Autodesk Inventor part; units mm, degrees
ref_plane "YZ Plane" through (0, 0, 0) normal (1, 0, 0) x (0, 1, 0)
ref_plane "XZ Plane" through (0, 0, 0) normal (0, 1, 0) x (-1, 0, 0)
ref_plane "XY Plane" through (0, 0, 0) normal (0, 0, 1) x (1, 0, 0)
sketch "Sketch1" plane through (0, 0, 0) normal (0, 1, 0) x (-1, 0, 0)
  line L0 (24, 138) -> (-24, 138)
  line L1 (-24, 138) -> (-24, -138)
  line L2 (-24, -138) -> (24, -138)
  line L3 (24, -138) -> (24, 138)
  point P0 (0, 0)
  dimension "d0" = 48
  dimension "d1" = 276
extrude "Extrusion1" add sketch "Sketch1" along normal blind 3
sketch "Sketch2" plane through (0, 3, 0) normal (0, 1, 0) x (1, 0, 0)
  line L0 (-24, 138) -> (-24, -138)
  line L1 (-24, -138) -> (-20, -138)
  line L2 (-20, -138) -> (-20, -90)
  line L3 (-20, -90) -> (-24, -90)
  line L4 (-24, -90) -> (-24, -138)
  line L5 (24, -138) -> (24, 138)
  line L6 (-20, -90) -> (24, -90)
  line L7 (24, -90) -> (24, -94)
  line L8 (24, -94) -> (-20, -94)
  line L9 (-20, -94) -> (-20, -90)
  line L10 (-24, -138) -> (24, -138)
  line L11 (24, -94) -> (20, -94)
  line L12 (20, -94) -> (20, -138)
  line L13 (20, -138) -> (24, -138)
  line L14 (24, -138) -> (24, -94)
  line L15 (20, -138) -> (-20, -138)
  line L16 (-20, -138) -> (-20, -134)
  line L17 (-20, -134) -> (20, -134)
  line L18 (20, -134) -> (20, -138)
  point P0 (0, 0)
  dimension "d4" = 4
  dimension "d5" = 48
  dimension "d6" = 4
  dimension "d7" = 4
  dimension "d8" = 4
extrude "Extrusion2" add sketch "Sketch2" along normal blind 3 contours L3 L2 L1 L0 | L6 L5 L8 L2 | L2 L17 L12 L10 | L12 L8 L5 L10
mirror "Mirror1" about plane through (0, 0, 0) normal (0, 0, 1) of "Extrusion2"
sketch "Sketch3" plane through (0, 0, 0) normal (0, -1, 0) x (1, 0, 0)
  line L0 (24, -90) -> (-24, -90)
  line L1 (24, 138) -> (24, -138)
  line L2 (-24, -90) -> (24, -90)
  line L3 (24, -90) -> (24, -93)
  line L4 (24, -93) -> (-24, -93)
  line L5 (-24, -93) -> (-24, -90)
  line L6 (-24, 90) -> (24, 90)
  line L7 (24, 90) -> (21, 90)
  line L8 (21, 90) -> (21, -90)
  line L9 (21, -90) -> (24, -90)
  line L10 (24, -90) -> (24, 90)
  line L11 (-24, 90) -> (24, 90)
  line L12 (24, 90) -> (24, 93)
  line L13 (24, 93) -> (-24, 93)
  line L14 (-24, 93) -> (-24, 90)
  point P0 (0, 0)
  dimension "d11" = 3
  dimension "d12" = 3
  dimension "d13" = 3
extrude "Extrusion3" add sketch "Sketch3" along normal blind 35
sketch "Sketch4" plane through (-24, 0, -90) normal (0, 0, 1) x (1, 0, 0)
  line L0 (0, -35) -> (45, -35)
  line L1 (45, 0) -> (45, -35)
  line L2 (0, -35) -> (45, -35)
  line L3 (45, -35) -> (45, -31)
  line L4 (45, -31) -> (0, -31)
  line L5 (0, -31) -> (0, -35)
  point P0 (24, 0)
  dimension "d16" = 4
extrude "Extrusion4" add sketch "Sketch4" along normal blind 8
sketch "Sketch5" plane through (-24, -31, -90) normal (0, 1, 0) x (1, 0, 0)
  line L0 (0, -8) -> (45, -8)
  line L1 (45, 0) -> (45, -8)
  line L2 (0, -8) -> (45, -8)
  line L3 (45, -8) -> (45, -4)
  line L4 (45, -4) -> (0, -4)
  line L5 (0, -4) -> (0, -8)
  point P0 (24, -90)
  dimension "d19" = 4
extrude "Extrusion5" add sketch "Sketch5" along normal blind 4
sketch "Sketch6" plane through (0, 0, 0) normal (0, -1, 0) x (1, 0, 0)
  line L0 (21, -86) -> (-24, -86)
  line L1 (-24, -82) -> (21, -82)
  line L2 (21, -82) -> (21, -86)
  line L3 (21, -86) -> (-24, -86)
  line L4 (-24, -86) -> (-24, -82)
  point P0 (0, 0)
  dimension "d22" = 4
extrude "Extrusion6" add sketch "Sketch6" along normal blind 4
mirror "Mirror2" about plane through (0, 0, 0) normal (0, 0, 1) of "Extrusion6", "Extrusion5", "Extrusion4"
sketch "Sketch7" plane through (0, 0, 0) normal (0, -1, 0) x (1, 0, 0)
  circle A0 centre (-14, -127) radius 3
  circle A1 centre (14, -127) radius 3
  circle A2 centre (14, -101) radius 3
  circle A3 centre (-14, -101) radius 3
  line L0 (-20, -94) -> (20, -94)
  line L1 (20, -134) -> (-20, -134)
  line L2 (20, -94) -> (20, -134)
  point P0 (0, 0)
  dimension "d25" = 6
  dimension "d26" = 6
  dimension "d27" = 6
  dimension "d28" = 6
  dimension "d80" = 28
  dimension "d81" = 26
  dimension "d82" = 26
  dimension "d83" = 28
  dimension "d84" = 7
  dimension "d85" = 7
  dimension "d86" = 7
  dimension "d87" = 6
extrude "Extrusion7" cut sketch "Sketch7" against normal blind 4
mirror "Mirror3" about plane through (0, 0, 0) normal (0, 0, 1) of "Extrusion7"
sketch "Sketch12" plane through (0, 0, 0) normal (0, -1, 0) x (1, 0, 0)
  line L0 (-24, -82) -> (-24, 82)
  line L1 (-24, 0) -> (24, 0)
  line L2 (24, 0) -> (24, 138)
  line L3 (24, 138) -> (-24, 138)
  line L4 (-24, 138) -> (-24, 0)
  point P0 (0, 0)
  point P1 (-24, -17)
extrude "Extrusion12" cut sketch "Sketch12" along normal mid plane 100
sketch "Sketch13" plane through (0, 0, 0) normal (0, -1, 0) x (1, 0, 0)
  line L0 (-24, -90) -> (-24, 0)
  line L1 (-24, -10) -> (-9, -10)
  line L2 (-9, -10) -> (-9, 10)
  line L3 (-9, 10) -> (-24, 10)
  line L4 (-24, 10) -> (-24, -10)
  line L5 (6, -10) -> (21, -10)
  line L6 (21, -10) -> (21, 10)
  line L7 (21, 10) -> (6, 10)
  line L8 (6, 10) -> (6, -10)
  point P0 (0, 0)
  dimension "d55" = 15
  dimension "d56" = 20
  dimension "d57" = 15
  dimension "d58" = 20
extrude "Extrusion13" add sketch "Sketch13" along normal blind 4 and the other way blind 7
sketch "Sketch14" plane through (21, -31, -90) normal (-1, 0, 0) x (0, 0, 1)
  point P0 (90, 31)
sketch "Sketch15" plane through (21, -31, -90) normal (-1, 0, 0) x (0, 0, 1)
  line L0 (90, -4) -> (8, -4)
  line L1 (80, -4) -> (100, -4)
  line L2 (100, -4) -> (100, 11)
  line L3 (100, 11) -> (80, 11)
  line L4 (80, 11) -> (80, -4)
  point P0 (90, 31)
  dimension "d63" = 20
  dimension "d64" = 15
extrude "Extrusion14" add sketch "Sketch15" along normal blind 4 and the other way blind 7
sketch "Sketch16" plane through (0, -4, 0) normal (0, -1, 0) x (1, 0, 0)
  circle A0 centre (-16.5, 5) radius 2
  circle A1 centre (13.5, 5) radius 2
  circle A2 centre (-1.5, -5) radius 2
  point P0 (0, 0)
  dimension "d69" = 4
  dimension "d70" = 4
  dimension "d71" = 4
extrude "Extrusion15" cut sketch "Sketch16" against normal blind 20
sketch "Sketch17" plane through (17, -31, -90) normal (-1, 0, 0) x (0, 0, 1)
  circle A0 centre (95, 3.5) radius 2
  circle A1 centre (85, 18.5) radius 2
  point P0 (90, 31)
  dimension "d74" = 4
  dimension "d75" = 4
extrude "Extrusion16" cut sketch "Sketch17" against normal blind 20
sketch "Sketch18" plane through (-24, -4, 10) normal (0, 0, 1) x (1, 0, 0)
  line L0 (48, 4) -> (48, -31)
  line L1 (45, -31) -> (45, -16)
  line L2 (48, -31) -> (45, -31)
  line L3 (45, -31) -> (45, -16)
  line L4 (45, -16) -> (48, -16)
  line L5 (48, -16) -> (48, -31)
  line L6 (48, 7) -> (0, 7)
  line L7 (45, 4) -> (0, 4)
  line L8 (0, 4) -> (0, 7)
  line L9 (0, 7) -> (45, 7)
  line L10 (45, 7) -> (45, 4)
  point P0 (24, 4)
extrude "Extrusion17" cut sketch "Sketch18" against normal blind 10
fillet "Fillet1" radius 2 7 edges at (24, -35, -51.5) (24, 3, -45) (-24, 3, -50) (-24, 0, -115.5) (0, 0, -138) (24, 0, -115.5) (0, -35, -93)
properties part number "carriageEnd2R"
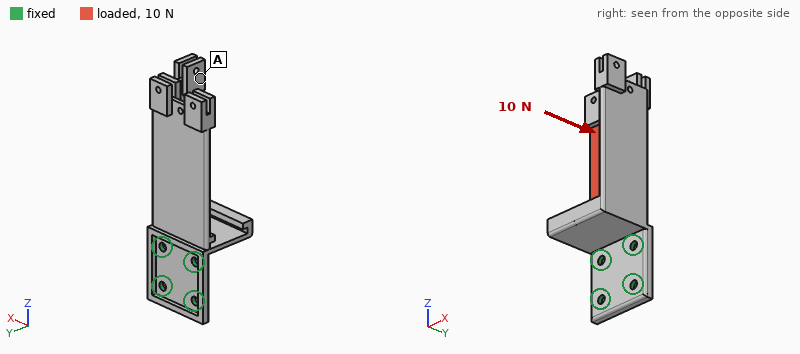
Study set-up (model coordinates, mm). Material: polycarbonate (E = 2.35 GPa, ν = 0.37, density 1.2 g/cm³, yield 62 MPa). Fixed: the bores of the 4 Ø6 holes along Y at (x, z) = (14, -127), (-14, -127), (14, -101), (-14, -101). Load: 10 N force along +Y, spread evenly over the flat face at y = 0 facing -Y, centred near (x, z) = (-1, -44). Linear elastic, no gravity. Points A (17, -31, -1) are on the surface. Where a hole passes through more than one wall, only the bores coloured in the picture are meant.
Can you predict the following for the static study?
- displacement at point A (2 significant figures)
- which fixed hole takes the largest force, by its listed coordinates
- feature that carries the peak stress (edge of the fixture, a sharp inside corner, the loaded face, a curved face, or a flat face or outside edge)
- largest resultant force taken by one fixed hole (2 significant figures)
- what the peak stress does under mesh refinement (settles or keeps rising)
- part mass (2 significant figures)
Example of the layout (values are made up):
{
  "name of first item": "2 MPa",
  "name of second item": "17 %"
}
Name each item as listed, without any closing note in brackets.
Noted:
{
  "displacement at point A": "1.4 mm",
  "which fixed hole takes the largest force, by its listed coordinates": "(14, -101)",
  "feature that carries the peak stress": "edge of the fixture",
  "largest resultant force taken by one fixed hole": "18 N",
  "what the peak stress does under mesh refinement": "keeps rising",
  "part mass": "55 g"
}
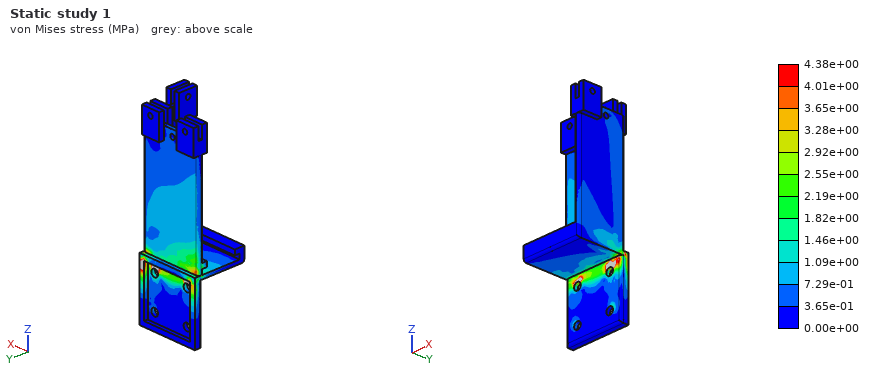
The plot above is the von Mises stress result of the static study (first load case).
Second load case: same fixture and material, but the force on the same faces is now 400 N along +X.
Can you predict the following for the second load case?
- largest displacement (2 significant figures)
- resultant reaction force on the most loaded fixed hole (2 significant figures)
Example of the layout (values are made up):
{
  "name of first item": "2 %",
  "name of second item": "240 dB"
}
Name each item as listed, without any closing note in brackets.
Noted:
{
  "largest displacement": "1.9 mm",
  "resultant reaction force on the most loaded fixed hole": "630 N"
}
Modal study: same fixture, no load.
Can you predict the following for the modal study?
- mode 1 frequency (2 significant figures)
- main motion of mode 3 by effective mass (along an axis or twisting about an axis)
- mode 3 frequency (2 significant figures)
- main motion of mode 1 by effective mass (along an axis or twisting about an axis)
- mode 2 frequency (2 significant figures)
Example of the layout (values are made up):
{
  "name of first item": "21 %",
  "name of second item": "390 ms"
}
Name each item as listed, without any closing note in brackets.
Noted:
{
  "mode 1 frequency": "71 Hz",
  "main motion of mode 3 by effective mass": "along X",
  "mode 3 frequency": "390 Hz",
  "main motion of mode 1 by effective mass": "along Y",
  "mode 2 frequency": "170 Hz"
}
